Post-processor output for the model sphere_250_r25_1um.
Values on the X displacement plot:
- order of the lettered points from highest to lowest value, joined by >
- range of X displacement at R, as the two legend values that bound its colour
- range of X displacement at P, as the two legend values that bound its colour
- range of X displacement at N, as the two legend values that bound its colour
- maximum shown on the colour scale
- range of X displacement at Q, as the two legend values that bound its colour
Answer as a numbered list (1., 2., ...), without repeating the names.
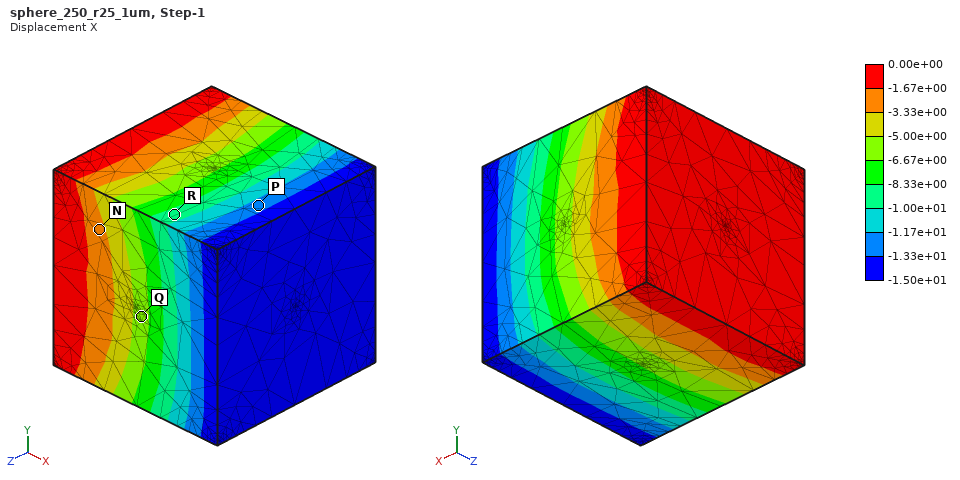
1. N > Q > R > P
2. -1.00e+01 to -8.33e+00
3. -1.33e+01 to -1.17e+01
4. -3.33e+00 to -1.67e+00
5. 0.00e+00
6. -6.67e+00 to -5.00e+00
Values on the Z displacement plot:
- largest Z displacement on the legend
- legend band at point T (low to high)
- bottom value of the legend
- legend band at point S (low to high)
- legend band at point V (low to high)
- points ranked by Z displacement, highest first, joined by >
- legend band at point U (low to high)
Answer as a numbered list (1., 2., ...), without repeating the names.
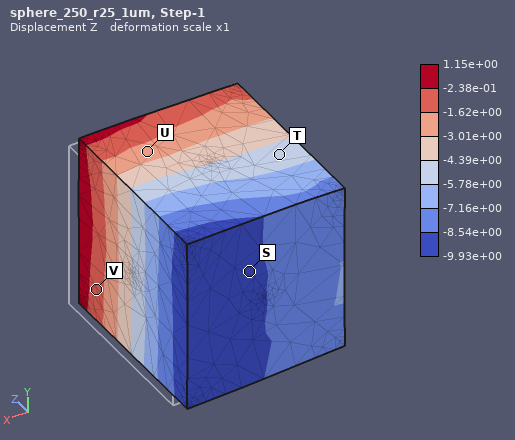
1. 1.15e+00
2. -5.78e+00 to -4.39e+00
3. -9.93e+00
4. -9.93e+00 to -8.54e+00
5. -1.62e+00 to -2.38e-01
6. V > U > T > S
7. -3.01e+00 to -1.62e+00
